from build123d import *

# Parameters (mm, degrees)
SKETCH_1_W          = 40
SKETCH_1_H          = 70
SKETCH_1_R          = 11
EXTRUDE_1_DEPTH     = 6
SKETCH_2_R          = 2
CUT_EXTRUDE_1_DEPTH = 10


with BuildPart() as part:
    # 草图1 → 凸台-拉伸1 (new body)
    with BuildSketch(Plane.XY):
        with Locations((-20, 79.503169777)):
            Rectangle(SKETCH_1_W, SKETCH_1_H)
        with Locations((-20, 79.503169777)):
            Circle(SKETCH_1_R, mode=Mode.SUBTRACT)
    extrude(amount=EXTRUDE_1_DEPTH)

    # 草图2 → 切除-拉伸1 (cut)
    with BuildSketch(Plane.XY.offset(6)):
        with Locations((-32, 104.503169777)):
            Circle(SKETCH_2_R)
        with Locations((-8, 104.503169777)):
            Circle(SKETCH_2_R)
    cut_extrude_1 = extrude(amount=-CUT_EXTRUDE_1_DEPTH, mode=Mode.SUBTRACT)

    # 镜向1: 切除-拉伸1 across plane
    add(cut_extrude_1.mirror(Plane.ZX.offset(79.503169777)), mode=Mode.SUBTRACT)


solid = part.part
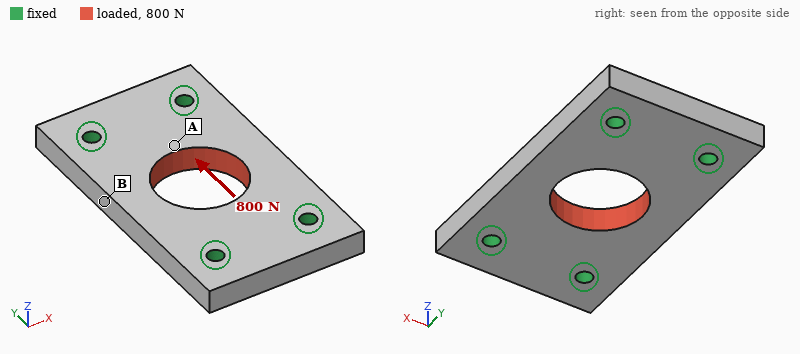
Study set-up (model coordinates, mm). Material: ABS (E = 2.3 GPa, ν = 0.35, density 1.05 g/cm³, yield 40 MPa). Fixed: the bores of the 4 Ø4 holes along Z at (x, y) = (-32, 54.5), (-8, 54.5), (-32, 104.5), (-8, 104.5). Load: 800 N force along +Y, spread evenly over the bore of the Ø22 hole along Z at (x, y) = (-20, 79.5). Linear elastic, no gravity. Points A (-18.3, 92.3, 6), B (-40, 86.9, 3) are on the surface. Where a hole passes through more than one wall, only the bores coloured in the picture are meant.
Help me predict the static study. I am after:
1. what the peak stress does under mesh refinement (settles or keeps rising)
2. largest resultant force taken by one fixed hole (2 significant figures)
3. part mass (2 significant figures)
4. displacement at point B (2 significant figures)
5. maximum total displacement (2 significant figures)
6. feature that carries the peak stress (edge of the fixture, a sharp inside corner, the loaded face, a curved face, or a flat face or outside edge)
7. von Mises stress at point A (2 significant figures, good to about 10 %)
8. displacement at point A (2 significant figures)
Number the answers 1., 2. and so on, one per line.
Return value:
1. keeps rising
2. 200 N
3. 15 g
4. 11 µm
5. 22 µm
6. edge of the fixture
7. 1.8 MPa
8. 15 µm
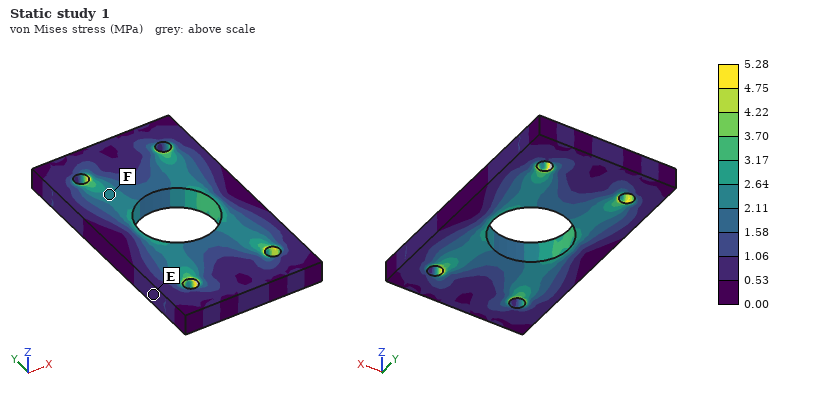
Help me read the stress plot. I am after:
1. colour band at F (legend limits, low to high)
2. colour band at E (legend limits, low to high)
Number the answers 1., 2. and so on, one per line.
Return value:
1. 2.11 to 2.64 MPa
2. 0.53 to 1.06 MPa
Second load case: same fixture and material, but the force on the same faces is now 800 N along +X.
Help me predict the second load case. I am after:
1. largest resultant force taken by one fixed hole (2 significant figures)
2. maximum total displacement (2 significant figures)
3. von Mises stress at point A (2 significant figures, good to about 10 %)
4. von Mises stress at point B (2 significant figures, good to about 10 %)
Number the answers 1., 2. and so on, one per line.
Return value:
1. 240 N
2. 69 µm
3. 5.0 MPa
4. 2.8 MPa
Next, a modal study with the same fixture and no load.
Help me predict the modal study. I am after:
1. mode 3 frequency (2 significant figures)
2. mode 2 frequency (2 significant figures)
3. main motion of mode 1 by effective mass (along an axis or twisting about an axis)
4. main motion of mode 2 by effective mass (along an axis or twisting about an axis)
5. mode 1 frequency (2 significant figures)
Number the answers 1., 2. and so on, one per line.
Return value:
1. 7200 Hz
2. 4000 Hz
3. along Z
4. twisting about Y
5. 3600 Hz
